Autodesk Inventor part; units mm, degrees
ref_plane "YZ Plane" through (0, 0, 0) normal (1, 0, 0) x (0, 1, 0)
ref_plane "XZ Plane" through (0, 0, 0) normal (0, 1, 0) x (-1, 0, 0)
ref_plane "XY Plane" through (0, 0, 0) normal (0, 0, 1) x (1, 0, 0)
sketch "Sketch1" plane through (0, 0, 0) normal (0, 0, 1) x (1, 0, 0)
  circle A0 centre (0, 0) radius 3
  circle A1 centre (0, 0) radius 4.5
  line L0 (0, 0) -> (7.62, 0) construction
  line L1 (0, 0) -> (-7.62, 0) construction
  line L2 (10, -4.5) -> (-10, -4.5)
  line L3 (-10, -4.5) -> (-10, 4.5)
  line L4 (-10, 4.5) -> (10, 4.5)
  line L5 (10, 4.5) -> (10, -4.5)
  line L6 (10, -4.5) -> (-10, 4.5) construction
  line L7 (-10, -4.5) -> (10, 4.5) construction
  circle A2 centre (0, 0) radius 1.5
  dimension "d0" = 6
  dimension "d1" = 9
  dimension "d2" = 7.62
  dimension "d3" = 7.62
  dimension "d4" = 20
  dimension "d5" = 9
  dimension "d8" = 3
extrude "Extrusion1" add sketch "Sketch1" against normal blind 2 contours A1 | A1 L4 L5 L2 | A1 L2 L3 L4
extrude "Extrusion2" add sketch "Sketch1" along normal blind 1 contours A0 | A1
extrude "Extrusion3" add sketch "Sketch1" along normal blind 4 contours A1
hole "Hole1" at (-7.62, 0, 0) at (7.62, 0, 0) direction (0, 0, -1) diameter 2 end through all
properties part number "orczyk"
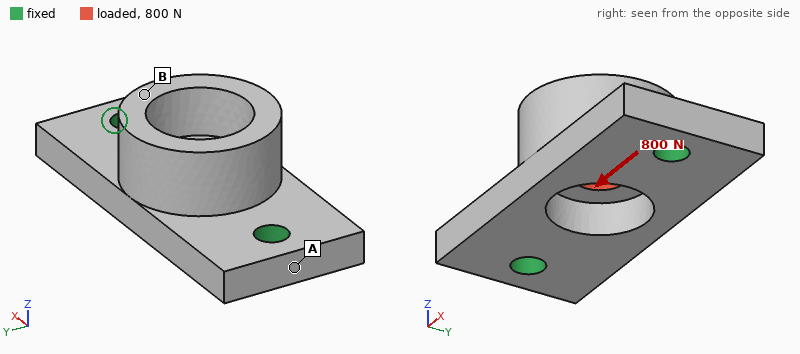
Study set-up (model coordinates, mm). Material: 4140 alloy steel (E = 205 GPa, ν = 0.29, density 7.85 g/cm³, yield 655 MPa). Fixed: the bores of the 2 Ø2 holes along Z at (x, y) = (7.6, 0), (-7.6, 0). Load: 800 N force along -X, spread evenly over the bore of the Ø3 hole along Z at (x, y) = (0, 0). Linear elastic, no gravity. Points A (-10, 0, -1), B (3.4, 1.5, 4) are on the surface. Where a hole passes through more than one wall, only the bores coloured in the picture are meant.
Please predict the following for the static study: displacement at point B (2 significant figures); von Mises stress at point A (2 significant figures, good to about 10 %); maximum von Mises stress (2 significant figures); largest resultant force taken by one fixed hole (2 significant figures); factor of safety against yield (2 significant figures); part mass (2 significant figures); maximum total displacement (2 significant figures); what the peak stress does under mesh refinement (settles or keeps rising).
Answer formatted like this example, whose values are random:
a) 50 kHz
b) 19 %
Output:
a) 1.4 µm
b) 26 MPa
c) 150 MPa
d) 410 N
e) 4.4
f) 3.6 g
g) 2.0 µm
h) settles
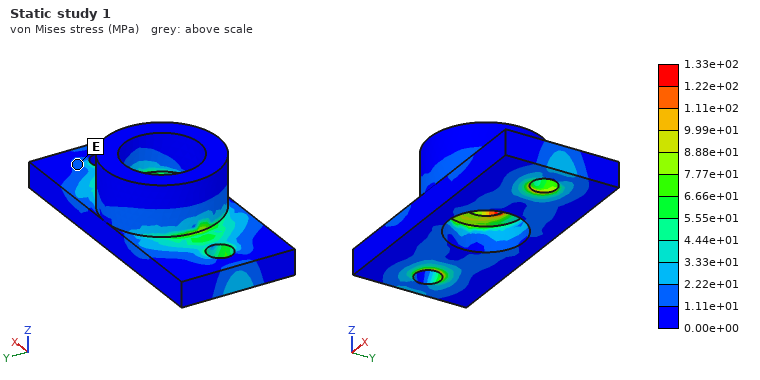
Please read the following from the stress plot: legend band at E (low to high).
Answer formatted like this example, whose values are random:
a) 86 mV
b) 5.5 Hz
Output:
a) 1.11e+01 to 2.22e+01 MPa
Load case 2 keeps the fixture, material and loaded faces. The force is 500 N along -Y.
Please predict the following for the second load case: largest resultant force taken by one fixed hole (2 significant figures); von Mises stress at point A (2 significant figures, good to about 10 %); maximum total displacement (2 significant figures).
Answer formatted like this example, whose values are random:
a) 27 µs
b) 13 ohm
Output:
a) 250 N
b) 23 MPa
c) 6.7 µm
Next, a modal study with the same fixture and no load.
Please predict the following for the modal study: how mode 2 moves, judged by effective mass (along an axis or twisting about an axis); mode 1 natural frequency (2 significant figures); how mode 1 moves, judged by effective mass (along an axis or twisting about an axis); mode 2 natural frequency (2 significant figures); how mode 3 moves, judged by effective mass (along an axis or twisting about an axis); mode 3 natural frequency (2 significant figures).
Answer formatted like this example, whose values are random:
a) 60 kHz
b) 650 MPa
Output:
a) along Z
b) 27 kHz
c) along Y
d) 40 kHz
e) along X
f) 65 kHz
